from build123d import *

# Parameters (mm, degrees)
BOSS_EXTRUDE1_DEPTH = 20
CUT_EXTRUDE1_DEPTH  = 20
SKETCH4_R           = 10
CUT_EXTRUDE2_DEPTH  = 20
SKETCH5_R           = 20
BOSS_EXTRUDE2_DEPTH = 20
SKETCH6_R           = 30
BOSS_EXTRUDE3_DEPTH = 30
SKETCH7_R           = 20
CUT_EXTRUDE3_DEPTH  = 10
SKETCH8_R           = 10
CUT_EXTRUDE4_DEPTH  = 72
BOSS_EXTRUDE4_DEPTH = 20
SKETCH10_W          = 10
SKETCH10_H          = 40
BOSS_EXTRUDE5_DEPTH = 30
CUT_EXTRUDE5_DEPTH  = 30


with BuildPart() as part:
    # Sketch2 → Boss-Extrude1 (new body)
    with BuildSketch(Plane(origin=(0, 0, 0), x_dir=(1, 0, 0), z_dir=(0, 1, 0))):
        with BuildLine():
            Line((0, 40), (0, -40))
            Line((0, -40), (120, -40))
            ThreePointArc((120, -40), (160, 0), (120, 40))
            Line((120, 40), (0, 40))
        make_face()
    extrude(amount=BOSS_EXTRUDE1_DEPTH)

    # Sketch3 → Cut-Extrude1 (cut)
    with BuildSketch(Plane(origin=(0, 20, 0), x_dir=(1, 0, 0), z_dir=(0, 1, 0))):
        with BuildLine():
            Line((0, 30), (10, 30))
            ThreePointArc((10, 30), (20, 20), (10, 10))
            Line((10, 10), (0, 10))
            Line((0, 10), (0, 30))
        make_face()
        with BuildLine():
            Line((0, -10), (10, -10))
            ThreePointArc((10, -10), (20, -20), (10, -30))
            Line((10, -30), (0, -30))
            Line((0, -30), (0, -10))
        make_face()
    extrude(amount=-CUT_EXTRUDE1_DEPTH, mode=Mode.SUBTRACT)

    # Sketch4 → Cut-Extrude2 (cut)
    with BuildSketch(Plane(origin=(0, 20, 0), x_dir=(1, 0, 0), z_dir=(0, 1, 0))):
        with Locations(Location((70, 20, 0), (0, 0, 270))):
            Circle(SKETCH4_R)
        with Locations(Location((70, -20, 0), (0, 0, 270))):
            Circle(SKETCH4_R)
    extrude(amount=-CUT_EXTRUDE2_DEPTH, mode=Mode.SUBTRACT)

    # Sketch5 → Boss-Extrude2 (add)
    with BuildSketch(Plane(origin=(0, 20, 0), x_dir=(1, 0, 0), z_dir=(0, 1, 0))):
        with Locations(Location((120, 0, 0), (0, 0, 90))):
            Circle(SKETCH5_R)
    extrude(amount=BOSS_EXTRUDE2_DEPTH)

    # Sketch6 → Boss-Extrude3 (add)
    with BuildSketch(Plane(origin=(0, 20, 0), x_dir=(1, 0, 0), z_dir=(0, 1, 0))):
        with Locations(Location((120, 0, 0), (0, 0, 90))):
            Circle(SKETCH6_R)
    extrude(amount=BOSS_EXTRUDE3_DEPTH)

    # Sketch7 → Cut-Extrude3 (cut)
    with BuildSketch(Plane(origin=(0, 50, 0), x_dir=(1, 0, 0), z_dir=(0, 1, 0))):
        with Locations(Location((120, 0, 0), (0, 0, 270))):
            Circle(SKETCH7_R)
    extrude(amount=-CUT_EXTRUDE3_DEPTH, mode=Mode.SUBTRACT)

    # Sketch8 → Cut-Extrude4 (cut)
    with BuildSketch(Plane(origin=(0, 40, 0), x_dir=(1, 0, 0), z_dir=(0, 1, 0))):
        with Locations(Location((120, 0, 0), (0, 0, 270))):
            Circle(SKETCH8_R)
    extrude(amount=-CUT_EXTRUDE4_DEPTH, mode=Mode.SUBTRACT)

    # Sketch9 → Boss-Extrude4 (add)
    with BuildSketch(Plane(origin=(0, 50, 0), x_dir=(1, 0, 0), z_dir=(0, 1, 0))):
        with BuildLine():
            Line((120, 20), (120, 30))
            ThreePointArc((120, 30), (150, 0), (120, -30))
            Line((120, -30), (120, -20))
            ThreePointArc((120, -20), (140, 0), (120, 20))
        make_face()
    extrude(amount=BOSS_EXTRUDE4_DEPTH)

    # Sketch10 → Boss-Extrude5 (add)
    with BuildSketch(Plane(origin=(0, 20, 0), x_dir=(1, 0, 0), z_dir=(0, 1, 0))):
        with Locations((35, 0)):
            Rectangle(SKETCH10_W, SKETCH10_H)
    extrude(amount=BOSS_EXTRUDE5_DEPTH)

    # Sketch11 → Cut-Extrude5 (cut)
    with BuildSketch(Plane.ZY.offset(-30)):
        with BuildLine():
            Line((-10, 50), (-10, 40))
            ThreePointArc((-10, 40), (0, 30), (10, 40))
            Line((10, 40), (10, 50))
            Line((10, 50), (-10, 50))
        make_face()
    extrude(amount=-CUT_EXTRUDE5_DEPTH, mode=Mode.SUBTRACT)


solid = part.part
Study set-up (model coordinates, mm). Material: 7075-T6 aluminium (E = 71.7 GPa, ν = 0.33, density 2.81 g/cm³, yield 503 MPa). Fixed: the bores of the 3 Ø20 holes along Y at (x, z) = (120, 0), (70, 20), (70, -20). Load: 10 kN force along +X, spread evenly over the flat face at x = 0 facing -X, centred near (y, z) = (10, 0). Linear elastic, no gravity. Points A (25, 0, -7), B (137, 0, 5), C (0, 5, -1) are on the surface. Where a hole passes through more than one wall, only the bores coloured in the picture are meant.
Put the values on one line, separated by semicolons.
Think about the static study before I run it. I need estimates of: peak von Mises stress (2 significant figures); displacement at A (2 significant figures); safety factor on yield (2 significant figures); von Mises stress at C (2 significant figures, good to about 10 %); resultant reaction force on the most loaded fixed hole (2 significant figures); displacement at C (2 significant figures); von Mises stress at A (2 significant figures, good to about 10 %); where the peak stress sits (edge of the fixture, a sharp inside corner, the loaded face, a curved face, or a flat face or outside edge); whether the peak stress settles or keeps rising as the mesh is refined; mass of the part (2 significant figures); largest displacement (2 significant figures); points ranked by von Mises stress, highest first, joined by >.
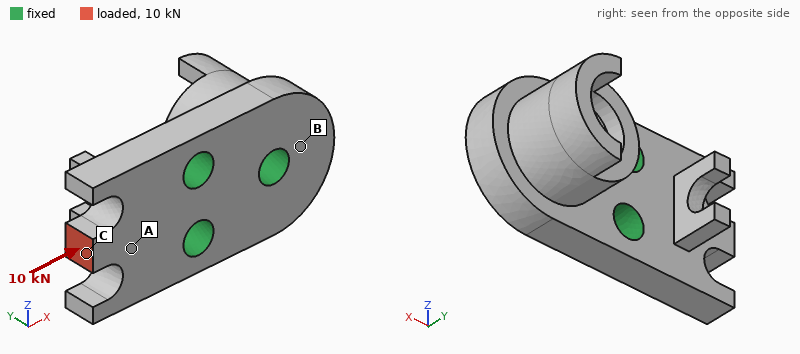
38 MPa; 6.2 µm; 13; 25 MPa; 5.2 kN; 13 µm; 17 MPa; a curved face; settles; 840 g; 14 µm; C > A > B
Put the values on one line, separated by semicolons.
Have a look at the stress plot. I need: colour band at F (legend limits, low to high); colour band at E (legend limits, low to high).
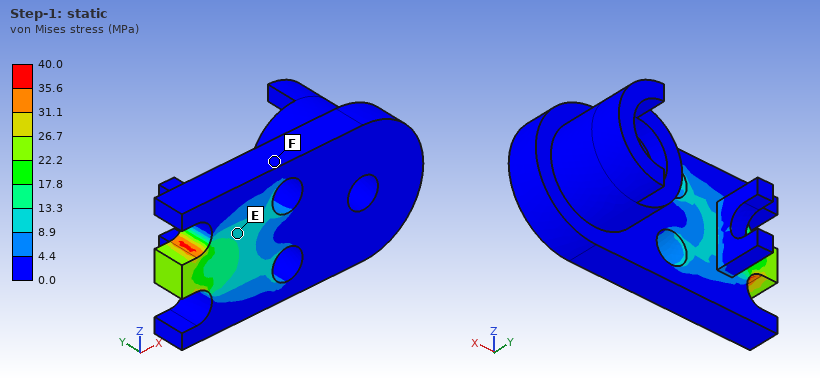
0.0 to 4.4 MPa; 8.9 to 13.3 MPa
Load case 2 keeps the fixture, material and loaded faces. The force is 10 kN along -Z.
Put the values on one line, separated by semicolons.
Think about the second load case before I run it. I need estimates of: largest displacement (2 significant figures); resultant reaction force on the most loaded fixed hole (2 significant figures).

84 µm; 13 kN
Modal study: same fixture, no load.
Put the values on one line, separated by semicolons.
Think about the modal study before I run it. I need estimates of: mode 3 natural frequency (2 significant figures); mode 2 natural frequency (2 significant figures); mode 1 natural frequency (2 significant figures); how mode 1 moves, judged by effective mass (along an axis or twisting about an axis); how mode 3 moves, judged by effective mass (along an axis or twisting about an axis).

9100 Hz; 6800 Hz; 4400 Hz; along Y; along Z
